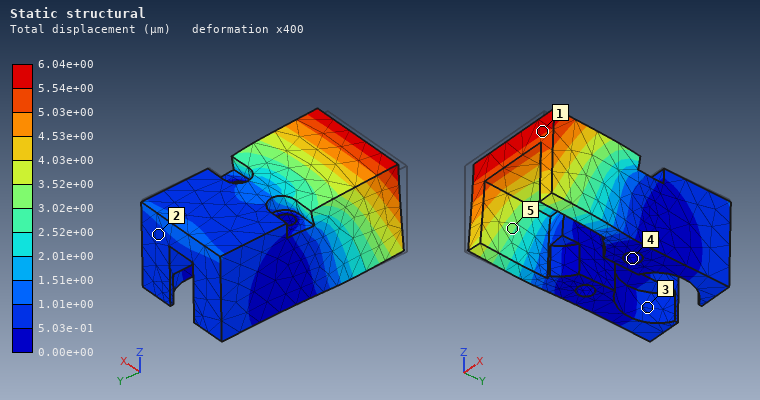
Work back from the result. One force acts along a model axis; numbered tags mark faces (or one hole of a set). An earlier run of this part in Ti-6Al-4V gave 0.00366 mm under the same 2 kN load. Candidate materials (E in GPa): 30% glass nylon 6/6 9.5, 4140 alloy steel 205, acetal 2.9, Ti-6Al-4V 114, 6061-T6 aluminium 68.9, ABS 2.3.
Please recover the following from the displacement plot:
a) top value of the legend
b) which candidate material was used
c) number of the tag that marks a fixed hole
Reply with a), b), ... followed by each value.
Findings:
a) 6.04e+00 µm
b) 6061-T6 aluminium
c) 4
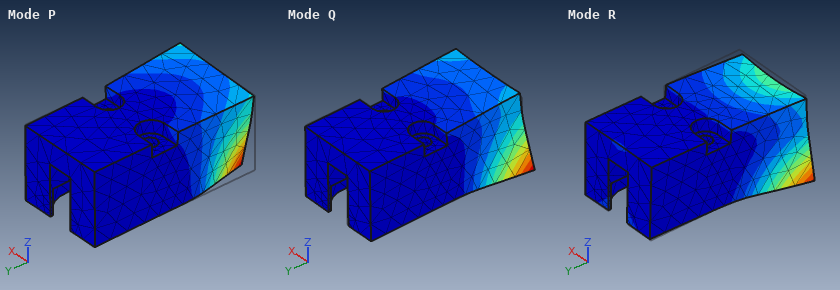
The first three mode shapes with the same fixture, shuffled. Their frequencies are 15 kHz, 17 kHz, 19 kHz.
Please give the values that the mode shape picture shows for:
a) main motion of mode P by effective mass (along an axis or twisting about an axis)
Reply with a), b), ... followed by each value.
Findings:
a) along X
